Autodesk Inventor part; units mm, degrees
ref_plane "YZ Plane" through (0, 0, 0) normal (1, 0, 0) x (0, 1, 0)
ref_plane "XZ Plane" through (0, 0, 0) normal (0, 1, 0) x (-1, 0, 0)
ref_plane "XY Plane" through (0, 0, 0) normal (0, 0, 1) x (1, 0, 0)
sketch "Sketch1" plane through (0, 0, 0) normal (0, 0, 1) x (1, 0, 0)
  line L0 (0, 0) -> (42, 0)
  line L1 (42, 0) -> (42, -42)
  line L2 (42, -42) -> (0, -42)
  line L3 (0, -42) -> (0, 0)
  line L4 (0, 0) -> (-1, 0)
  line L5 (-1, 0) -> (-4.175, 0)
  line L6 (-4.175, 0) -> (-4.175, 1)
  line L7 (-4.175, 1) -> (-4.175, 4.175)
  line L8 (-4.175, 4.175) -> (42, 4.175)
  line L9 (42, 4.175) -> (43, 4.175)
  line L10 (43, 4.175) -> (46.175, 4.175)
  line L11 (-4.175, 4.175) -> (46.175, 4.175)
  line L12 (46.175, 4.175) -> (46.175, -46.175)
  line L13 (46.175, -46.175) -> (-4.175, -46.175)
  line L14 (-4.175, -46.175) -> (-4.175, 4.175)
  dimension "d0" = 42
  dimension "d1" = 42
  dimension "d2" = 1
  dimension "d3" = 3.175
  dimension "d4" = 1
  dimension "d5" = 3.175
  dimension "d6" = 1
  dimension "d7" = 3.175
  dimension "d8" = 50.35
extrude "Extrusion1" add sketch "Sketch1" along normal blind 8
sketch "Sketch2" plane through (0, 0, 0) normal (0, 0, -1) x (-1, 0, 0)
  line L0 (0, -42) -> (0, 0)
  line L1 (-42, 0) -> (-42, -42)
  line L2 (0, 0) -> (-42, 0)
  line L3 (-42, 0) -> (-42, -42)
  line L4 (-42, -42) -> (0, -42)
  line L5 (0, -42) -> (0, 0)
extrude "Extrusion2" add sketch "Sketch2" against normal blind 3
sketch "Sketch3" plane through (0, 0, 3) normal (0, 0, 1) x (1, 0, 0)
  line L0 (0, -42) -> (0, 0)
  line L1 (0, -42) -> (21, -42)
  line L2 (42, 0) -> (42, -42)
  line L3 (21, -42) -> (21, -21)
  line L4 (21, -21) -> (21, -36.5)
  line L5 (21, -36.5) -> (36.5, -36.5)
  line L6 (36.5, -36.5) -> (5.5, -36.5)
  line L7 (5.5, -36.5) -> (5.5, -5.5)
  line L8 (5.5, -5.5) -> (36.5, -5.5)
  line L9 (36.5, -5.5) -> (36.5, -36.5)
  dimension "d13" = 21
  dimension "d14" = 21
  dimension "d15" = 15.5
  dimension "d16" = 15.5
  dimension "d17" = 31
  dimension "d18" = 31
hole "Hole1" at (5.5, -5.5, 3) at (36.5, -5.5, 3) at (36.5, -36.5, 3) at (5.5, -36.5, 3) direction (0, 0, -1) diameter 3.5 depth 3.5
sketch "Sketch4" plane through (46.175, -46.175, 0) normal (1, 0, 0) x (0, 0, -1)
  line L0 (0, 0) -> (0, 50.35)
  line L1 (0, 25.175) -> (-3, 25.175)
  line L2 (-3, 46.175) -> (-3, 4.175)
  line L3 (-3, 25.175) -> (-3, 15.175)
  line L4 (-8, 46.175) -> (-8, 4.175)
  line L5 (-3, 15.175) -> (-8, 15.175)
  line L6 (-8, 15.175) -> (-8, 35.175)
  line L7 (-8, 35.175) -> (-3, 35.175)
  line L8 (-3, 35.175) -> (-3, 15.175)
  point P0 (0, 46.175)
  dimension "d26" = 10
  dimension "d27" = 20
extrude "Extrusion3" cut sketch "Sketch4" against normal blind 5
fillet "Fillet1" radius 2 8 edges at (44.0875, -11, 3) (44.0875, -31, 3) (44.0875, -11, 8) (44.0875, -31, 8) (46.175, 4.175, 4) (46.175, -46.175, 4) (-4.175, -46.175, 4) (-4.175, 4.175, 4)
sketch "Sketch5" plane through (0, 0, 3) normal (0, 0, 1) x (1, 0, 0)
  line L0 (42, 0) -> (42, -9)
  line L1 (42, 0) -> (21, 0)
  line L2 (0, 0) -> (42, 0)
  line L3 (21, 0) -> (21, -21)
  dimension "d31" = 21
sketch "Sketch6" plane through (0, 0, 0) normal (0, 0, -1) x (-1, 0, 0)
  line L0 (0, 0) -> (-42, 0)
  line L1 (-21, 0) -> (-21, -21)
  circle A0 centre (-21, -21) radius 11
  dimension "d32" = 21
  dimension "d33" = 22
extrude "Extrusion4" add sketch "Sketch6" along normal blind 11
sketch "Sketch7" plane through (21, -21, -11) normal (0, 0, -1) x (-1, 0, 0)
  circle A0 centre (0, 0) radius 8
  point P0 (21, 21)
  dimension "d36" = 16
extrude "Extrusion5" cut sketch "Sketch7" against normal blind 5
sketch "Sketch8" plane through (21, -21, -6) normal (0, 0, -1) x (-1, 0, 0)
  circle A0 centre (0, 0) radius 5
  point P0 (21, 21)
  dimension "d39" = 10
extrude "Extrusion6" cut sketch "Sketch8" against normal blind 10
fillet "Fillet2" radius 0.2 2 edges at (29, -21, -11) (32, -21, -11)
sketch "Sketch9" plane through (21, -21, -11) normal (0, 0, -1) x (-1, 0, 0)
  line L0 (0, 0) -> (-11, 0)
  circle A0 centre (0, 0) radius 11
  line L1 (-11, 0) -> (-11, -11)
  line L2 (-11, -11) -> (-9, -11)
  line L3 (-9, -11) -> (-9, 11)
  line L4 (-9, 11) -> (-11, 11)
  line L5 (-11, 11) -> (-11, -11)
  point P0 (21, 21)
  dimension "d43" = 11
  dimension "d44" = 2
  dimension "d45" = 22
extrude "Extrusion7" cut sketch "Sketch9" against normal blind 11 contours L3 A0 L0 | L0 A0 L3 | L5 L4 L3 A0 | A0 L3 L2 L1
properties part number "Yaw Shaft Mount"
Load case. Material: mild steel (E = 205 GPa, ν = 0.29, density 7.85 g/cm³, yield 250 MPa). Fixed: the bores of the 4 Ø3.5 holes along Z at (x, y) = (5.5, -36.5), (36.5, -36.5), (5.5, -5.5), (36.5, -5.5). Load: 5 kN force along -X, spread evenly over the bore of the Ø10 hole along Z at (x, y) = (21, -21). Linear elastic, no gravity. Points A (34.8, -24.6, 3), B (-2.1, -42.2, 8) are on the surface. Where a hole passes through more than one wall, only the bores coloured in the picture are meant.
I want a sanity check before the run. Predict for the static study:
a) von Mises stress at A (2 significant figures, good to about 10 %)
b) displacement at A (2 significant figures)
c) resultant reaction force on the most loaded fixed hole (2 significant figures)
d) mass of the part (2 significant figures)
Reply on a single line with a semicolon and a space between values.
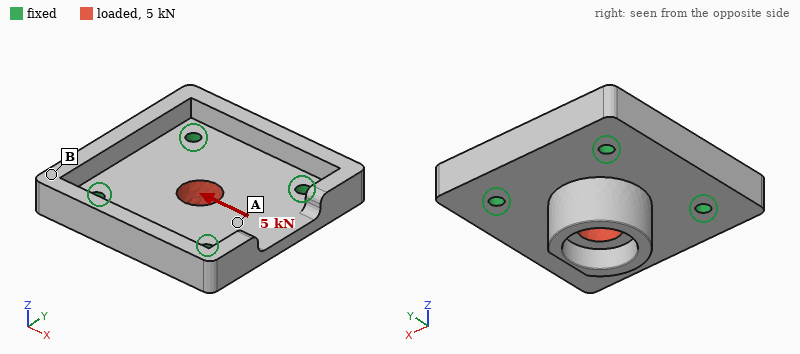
22 MPa; 5.6 µm; 1.3 kN; 100 g
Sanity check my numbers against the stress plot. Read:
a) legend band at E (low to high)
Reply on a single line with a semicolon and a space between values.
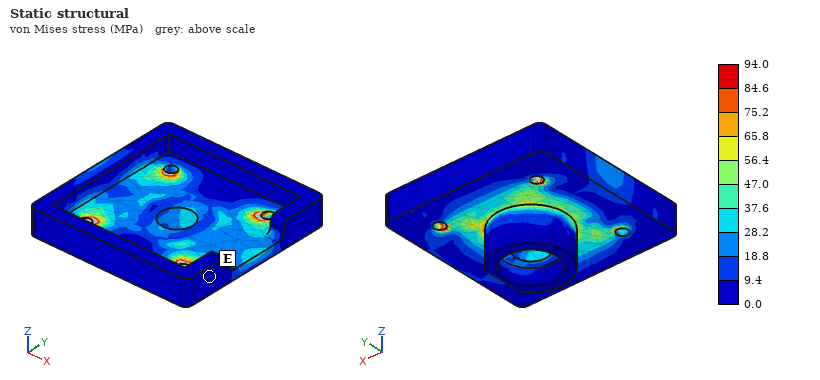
0.0 to 9.4 MPa
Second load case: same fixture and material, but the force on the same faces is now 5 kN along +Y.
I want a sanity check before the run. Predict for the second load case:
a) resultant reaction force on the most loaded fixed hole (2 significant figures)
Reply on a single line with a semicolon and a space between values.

1.3 kN
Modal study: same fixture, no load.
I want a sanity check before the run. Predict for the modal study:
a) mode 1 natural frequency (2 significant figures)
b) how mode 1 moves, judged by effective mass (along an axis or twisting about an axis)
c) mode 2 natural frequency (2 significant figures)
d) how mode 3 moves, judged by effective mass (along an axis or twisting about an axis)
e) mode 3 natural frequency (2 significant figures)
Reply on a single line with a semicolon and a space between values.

11 kHz; along Z; 13 kHz; twisting about X; 14 kHz
